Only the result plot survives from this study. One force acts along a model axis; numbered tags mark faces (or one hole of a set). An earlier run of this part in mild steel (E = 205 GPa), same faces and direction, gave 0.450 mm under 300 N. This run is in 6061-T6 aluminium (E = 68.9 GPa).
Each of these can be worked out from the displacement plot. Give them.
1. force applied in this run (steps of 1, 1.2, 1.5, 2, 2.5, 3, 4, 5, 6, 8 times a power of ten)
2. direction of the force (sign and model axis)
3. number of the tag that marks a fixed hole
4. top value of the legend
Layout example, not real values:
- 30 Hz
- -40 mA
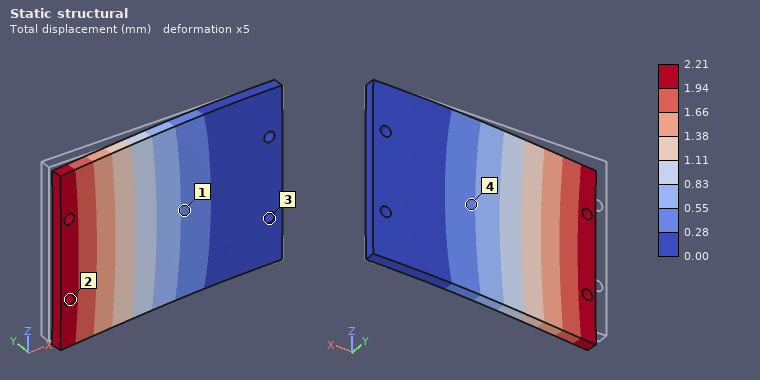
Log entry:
- 500 N
- -Y
- 3
- 2.21 mm
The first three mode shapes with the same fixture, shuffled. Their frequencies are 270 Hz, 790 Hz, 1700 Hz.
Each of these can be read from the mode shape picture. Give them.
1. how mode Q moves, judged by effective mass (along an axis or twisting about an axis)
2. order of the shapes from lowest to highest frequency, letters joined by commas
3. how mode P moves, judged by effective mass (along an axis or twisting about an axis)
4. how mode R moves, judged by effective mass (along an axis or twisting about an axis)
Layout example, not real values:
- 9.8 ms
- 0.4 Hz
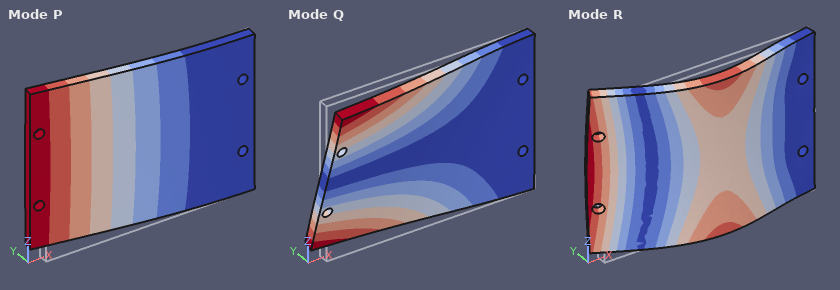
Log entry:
- twisting about X
- P, Q, R
- along Y
- along Y
